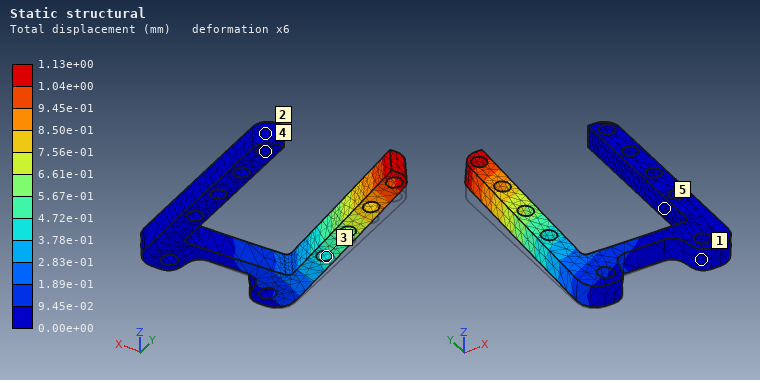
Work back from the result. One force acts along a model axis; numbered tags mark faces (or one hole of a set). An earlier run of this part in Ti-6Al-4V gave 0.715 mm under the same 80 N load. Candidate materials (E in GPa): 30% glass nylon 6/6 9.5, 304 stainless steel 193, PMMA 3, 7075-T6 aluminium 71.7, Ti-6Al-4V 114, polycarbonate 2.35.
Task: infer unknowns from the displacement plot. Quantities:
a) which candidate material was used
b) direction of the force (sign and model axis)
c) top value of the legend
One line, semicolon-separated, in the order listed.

7075-T6 aluminium; +Z; 1.13e+00 mm
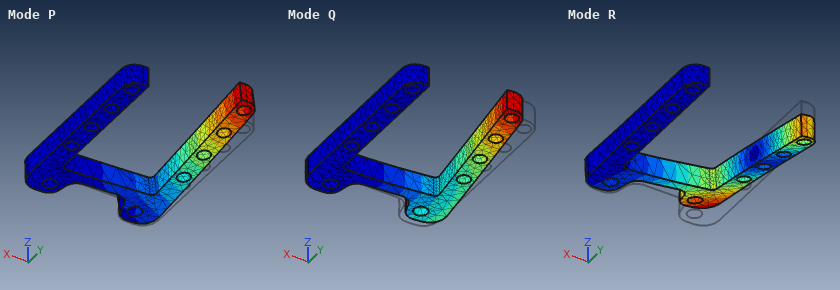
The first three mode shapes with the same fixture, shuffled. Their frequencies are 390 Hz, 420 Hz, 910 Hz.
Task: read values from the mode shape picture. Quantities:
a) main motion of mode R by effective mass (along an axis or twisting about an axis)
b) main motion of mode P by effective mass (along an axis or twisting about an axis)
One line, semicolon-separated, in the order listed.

along Z; along Z
